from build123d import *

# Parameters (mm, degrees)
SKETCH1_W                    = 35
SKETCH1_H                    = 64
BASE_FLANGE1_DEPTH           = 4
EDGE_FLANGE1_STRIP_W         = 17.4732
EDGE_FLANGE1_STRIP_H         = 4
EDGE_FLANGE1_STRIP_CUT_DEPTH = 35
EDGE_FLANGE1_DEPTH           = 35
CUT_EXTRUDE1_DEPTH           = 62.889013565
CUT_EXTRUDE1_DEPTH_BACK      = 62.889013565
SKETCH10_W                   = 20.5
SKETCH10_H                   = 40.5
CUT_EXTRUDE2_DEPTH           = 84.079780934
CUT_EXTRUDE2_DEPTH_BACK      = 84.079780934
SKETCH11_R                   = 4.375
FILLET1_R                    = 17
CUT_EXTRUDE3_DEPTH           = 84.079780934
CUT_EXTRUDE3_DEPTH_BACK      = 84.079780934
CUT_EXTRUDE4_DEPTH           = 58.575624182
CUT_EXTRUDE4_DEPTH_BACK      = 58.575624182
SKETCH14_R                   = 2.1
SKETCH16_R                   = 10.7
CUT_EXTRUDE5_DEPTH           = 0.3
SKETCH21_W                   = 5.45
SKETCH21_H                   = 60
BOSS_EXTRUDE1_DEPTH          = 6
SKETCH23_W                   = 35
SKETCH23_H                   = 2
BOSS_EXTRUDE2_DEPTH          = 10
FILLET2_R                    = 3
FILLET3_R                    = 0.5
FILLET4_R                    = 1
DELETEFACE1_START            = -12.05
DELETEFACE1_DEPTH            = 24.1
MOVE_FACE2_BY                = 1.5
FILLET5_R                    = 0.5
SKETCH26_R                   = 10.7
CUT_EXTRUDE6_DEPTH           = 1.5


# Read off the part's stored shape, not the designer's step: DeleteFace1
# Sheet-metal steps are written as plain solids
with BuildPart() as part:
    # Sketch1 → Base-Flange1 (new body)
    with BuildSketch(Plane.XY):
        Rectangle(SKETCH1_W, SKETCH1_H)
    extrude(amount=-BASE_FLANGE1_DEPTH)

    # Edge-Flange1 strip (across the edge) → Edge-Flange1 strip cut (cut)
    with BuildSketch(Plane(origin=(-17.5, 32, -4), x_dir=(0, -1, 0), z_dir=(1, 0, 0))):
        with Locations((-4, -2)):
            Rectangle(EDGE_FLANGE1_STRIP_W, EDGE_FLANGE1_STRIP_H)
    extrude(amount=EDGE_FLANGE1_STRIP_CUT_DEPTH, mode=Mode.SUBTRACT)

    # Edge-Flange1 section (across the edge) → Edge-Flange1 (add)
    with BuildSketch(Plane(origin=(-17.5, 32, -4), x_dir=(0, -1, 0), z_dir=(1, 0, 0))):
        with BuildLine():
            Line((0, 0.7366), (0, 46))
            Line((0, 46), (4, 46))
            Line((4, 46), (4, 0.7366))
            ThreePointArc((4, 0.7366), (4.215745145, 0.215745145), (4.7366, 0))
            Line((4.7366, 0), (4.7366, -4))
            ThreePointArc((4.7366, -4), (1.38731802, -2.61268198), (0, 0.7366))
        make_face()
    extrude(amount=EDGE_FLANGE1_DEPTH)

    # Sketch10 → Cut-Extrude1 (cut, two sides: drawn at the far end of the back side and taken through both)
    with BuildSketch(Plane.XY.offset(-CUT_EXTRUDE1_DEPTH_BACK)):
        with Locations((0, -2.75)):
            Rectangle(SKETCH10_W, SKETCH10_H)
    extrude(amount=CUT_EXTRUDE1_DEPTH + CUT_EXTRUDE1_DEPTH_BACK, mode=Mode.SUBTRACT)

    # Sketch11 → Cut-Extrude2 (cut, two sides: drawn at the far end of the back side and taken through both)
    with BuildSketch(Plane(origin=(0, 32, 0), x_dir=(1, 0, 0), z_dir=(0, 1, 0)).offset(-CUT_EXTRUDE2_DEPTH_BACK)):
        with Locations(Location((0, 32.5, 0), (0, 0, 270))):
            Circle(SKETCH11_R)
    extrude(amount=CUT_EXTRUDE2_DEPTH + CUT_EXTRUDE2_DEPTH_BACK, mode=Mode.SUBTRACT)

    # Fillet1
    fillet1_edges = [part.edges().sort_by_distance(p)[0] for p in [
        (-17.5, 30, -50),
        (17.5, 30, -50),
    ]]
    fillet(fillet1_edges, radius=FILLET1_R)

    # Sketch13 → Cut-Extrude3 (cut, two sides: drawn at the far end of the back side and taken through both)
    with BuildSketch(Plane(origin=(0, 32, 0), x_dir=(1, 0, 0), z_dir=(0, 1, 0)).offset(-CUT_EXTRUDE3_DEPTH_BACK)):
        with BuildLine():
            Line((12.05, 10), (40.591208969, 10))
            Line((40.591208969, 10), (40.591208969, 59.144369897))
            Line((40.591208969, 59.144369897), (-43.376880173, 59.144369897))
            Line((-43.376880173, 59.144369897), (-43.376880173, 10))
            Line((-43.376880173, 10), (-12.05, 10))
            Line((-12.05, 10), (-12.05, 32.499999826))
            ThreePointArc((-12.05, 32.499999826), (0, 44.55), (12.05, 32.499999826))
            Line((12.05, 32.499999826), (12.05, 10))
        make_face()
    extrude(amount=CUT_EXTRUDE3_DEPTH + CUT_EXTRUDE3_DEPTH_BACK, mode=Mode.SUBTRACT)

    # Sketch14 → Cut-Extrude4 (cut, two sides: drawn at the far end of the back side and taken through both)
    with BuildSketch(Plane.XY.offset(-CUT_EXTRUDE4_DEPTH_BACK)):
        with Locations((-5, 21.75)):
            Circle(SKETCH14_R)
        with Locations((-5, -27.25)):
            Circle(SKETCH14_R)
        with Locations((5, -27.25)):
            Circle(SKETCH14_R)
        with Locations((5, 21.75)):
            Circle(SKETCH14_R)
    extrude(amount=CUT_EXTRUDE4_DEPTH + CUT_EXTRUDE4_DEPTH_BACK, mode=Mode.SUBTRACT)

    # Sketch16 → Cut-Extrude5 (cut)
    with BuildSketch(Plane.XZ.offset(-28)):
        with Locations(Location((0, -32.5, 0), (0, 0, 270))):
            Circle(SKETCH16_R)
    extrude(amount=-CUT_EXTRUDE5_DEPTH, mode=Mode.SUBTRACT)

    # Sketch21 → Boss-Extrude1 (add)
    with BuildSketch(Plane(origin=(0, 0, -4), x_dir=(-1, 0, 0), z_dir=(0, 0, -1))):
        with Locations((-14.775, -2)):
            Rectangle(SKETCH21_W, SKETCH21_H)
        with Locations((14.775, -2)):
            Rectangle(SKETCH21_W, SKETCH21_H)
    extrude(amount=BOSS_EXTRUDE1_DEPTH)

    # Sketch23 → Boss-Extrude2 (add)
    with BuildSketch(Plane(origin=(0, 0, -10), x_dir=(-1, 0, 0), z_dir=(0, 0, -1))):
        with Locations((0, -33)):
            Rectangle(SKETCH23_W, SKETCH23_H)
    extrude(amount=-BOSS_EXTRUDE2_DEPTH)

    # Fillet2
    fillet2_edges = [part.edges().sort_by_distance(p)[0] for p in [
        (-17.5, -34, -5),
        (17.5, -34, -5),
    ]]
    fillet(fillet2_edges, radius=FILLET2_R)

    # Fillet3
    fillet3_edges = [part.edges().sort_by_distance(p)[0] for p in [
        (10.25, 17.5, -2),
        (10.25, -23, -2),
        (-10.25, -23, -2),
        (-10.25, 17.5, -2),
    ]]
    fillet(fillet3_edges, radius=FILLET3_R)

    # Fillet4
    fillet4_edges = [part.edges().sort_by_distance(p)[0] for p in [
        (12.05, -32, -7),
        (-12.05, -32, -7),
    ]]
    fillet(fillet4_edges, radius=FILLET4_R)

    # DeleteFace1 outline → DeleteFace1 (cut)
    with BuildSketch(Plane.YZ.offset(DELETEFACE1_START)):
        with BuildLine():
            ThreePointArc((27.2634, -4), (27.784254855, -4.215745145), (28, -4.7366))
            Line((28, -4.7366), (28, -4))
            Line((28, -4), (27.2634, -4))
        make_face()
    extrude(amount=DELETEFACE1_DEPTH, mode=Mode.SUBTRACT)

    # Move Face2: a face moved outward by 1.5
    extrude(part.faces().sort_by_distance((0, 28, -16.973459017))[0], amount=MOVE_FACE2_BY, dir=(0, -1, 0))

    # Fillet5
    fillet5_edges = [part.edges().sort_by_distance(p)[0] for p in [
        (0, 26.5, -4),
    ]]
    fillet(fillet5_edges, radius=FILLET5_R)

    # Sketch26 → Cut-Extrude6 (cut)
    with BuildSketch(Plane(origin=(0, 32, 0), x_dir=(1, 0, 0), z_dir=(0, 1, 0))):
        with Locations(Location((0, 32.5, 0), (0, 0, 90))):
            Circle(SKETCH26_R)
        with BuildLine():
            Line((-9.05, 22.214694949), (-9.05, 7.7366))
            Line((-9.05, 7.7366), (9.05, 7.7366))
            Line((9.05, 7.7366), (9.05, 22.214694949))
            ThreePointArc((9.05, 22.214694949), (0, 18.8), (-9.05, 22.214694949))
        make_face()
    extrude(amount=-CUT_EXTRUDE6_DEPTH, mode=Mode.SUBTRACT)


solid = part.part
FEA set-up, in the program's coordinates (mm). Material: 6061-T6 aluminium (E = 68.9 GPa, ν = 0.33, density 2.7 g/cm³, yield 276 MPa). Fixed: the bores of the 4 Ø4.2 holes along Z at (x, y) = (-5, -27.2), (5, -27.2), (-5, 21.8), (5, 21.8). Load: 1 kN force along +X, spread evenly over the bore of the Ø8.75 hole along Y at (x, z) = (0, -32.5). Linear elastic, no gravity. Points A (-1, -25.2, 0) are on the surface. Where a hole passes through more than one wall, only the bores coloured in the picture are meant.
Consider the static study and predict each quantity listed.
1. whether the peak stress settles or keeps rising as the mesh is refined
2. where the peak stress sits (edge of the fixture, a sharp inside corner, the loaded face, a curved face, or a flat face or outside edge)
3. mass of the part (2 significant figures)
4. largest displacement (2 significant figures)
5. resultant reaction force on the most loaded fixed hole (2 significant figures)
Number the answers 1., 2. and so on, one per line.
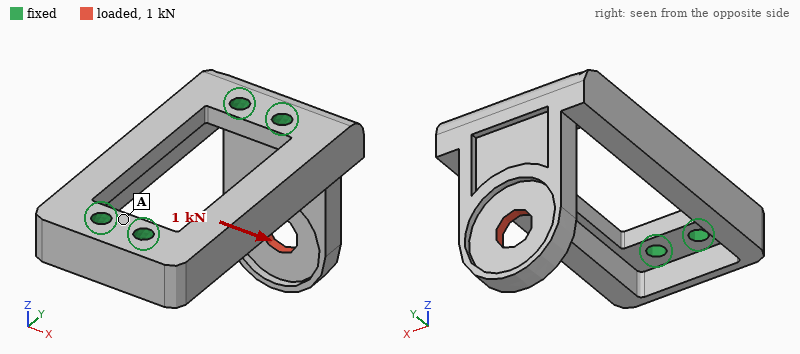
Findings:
1. keeps rising
2. edge of the fixture
3. 36 g
4. 0.18 mm
5. 2.0 kN
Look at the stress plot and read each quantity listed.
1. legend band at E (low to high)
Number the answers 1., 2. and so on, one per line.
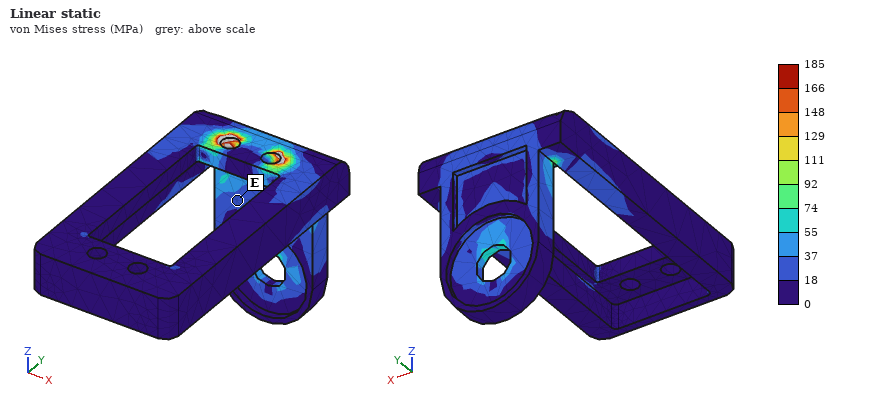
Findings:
1. 18 to 37 MPa
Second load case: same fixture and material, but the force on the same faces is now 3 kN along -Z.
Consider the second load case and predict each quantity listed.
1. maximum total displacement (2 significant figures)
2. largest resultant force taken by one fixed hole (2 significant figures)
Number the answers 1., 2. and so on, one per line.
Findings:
1. 0.20 mm
2. 1.6 kN
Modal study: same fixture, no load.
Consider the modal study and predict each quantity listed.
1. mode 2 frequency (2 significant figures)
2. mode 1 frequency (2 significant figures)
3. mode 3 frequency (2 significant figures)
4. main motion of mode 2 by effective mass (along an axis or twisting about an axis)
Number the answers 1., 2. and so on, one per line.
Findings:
1. 6100 Hz
2. 2900 Hz
3. 7800 Hz
4. along X
